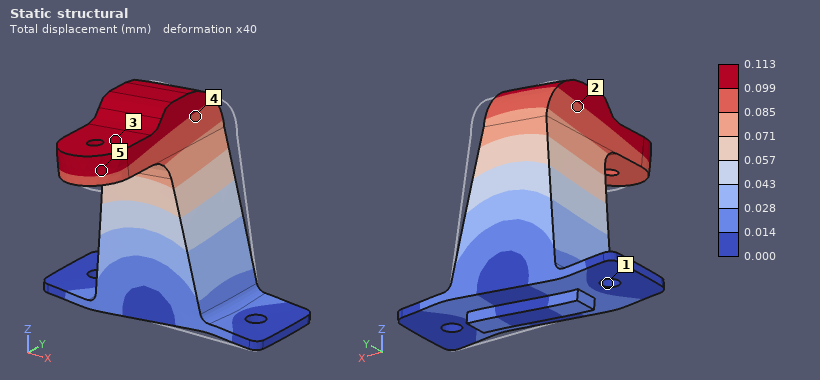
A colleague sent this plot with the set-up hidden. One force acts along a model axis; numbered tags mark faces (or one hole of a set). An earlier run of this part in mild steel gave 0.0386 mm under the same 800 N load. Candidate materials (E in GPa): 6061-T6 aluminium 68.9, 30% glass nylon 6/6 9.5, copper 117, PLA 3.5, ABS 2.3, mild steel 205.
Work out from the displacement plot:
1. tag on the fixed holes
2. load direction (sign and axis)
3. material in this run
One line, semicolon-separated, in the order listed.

1; -X; 6061-T6 aluminium
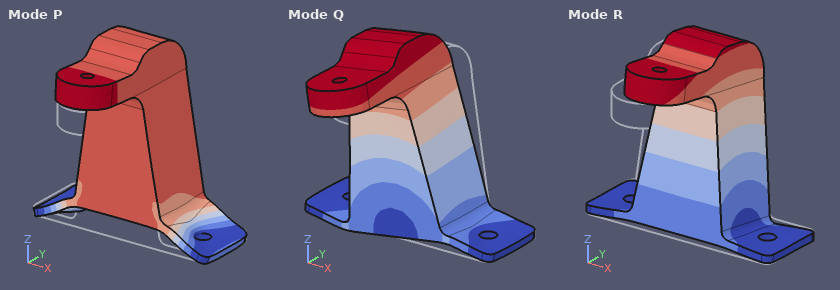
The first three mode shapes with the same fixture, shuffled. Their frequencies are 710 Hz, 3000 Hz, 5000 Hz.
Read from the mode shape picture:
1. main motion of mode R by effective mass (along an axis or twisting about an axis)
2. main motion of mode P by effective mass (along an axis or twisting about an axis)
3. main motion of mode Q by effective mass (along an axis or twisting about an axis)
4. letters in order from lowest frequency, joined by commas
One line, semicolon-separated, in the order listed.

along Y; along Z; along X; R, Q, P
